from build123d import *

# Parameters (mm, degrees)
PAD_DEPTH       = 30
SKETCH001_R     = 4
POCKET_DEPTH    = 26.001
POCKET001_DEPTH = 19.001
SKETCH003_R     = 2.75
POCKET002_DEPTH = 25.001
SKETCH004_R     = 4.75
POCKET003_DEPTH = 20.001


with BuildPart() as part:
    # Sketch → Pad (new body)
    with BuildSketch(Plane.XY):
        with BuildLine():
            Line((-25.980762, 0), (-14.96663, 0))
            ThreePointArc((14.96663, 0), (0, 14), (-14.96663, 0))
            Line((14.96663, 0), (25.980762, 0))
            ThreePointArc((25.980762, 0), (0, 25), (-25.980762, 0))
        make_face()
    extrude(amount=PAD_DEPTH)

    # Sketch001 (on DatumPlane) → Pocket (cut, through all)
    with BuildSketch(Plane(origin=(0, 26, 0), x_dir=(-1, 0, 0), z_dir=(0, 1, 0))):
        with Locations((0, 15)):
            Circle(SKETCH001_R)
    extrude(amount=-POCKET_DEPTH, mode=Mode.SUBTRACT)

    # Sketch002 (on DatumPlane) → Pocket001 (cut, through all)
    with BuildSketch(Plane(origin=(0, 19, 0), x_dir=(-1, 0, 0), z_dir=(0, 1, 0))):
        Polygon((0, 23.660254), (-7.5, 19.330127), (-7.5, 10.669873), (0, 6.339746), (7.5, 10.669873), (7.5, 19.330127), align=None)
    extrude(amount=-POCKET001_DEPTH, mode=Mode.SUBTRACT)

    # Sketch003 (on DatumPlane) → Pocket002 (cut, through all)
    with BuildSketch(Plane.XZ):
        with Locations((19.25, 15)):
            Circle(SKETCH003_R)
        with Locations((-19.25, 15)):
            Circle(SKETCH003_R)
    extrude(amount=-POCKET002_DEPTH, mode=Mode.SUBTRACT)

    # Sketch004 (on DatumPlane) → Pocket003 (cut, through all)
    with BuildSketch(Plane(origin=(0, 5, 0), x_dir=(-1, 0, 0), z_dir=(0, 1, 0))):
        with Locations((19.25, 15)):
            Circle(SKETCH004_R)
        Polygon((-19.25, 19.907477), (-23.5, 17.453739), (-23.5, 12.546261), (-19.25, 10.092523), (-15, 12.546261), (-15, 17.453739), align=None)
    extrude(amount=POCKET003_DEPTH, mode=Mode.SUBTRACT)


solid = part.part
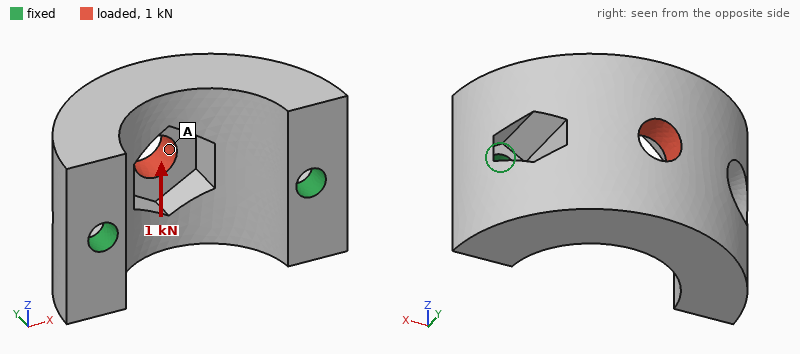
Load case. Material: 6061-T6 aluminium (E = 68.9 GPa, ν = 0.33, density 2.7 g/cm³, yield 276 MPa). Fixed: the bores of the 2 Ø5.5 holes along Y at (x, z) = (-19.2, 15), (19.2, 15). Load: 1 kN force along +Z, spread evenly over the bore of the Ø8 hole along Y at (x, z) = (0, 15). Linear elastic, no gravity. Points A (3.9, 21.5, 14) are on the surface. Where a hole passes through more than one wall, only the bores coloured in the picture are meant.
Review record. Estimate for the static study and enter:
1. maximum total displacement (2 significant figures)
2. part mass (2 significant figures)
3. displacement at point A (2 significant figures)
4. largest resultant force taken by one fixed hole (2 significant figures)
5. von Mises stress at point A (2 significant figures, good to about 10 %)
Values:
40 µm
47 g
29 µm
500 N
13 MPa
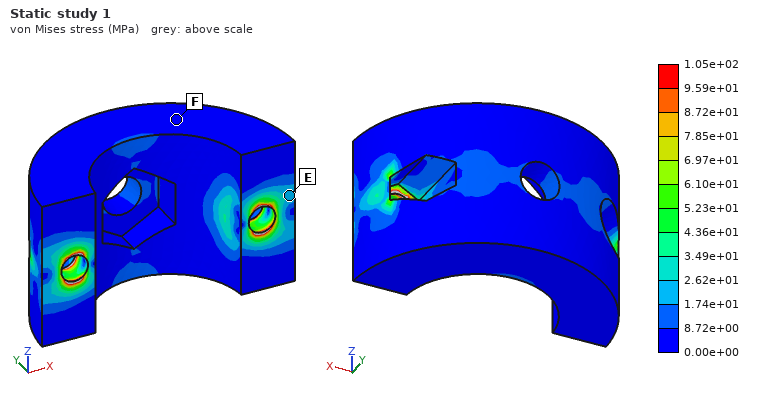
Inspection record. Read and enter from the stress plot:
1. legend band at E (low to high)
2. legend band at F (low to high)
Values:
1.74e+01 to 2.62e+01 MPa
0.00e+00 to 8.72e+00 MPa
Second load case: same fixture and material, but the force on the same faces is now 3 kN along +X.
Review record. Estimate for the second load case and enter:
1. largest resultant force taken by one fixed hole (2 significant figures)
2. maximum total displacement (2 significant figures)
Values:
2.0 kN
18 µm
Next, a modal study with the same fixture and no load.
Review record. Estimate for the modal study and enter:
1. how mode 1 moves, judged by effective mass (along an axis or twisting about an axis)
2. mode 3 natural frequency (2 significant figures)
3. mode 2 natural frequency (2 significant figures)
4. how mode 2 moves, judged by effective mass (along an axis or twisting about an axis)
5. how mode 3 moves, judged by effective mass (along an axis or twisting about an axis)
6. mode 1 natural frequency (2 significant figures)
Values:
along Z
15 kHz
14 kHz
along X
twisting about Y
5700 Hz
